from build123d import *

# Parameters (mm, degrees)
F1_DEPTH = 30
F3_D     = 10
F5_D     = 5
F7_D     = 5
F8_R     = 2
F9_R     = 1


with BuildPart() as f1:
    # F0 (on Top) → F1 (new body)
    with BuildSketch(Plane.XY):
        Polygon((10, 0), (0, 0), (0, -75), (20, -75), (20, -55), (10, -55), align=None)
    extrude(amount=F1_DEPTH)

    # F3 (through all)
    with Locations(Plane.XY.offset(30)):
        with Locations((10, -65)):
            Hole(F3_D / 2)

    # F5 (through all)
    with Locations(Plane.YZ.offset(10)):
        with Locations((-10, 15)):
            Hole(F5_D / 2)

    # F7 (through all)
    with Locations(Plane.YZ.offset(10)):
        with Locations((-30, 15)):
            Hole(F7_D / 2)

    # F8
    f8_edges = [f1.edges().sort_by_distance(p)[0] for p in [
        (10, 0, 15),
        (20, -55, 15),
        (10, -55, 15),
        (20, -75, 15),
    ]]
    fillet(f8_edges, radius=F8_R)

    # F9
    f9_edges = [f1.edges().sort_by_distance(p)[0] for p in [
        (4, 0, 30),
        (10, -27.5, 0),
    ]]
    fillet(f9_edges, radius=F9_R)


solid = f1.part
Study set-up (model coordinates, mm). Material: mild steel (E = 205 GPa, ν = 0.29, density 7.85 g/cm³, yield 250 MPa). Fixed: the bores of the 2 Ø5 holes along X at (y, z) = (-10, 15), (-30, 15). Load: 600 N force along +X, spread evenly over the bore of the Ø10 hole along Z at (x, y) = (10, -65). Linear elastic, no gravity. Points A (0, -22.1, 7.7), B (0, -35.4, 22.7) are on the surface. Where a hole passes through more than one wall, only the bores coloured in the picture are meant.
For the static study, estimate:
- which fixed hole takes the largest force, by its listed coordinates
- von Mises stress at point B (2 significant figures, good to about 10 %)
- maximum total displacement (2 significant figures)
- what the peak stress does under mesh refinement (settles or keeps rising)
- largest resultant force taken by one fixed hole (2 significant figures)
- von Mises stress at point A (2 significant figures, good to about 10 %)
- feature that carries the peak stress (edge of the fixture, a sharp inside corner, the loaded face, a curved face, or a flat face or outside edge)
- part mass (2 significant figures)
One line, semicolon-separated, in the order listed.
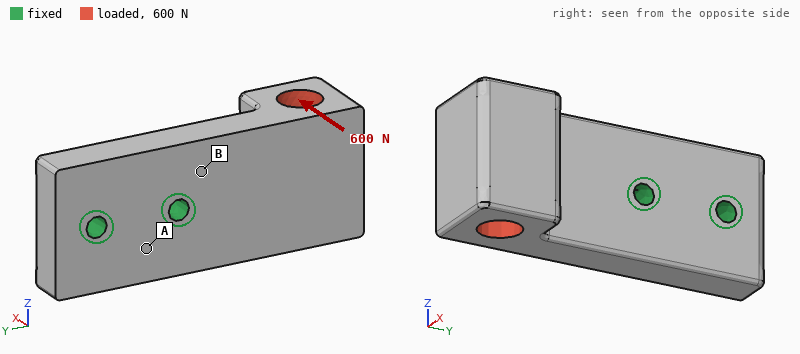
(-30, 15); 29 MPa; 29 µm; keeps rising; 960 N; 8.4 MPa; edge of the fixture; 200 g
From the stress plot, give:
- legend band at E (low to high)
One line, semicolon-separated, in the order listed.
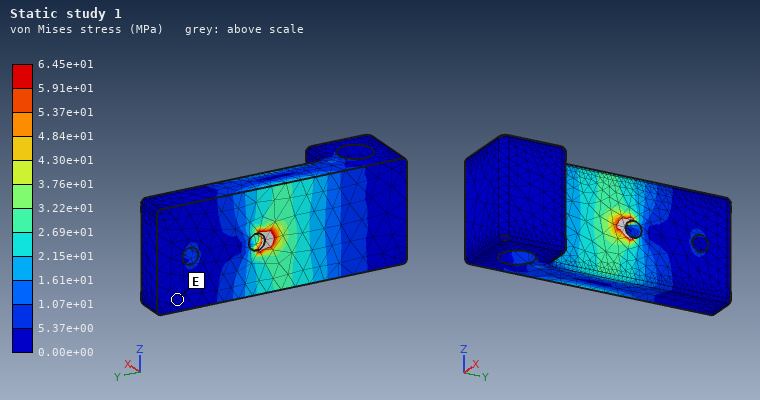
0.00e+00 to 5.37e+00 MPa
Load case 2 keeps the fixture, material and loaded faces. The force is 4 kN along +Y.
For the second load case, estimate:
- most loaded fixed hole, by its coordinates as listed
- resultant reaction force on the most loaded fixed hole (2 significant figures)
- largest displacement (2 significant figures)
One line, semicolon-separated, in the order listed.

(-30, 15); 3.2 kN; 42 µm
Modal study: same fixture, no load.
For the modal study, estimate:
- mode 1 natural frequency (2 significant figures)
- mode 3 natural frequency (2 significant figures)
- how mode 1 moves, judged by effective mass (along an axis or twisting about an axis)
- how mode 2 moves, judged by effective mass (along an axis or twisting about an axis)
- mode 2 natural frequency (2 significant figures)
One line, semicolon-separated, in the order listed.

2900 Hz; 7900 Hz; along X; along Z; 5200 Hz
